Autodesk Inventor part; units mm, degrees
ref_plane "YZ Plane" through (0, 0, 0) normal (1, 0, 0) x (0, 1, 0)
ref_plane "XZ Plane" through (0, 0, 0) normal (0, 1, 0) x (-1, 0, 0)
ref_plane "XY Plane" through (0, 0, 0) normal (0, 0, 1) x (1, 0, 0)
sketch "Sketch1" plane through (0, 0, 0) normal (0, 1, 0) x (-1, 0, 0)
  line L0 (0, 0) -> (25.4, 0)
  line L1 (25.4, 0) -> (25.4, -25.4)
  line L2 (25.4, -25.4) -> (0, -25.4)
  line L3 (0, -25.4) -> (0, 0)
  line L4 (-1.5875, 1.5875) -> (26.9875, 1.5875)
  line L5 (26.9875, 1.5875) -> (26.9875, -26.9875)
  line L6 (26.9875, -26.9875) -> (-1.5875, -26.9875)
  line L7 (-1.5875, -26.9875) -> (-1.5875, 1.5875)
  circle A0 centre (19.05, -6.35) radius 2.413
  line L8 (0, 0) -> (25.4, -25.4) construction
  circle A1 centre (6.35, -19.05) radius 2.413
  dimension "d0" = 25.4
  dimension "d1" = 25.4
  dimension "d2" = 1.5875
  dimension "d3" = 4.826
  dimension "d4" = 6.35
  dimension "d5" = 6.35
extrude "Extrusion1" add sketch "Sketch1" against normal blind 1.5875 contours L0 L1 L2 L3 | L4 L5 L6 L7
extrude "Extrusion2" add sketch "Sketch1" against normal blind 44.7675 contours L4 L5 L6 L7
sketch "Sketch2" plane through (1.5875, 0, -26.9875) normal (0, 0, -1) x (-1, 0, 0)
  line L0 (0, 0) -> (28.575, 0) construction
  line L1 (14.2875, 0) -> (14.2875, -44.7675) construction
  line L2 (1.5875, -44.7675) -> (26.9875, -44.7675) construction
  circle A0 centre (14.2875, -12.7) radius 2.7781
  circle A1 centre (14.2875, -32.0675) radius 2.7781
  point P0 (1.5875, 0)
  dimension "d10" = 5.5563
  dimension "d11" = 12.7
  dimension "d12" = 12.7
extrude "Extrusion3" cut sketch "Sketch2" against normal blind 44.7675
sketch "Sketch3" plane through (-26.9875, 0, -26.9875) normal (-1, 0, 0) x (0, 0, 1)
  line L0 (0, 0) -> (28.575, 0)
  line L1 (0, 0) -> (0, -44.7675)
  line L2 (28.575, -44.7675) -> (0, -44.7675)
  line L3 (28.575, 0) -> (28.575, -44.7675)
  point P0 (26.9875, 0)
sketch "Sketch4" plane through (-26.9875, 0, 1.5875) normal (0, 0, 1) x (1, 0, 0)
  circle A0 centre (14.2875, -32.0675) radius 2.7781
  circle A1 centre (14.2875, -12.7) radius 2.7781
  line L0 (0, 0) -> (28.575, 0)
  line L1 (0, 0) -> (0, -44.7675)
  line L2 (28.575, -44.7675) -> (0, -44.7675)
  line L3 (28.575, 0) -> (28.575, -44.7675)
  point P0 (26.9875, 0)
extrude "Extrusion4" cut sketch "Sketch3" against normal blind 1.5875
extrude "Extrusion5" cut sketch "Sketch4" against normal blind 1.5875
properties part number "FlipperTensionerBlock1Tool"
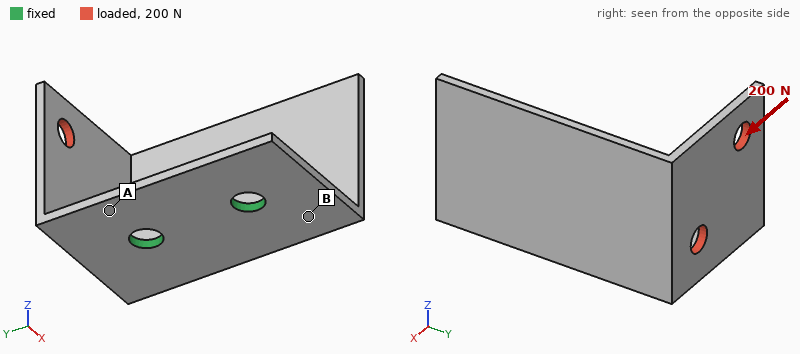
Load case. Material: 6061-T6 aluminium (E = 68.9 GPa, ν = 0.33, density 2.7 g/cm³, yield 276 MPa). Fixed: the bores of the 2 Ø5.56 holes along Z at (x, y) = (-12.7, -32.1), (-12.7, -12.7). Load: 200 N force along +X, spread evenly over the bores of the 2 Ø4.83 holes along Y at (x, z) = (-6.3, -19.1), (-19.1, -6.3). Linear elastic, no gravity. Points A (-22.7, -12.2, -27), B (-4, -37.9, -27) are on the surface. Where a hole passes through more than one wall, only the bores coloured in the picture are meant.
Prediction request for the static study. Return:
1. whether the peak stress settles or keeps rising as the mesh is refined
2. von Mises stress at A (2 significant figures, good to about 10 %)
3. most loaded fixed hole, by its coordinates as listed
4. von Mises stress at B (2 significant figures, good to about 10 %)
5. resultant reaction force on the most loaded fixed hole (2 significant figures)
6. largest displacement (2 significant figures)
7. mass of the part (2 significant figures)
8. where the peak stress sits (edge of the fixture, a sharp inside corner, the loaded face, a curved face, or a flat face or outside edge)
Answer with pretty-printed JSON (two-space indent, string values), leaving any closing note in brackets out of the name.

{
  "whether the peak stress settles or keeps rising as the mesh is refined": "keeps rising",
  "von Mises stress at A": "86 MPa",
  "most loaded fixed hole, by its coordinates as listed": "(-12.7, -12.7)",
  "von Mises stress at B": "35 MPa",
  "resultant reaction force on the most loaded fixed hole": "270 N",
  "largest displacement": "0.45 mm",
  "mass of the part": "12 g",
  "where the peak stress sits": "edge of the fixture"
}
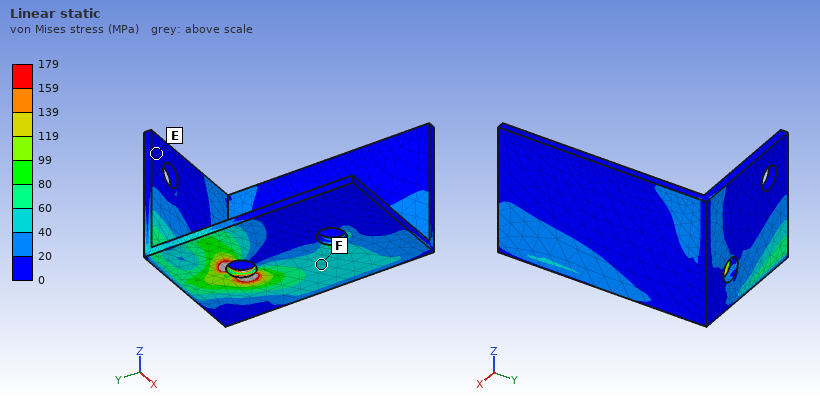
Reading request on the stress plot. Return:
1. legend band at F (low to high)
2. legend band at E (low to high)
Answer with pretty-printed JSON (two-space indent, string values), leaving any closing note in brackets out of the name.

{
  "legend band at F": "40 to 60 MPa",
  "legend band at E": "0 to 20 MPa"
}
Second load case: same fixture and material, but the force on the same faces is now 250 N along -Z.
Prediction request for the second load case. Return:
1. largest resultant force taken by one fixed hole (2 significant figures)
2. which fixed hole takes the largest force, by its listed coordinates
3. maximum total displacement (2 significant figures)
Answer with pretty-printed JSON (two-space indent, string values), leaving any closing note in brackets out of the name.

{
  "largest resultant force taken by one fixed hole": "300 N",
  "which fixed hole takes the largest force, by its listed coordinates": "(-12.7, -12.7)",
  "maximum total displacement": "0.24 mm"
}
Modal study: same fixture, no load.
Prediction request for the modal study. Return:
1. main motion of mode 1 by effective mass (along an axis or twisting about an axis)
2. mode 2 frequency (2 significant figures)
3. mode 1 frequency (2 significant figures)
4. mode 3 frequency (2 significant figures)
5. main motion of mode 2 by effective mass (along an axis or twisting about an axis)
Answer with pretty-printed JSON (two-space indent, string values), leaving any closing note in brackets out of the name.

{
  "main motion of mode 1 by effective mass": "along X",
  "mode 2 frequency": "1800 Hz",
  "mode 1 frequency": "1400 Hz",
  "mode 3 frequency": "2800 Hz",
  "main motion of mode 2 by effective mass": "along Y"
}
